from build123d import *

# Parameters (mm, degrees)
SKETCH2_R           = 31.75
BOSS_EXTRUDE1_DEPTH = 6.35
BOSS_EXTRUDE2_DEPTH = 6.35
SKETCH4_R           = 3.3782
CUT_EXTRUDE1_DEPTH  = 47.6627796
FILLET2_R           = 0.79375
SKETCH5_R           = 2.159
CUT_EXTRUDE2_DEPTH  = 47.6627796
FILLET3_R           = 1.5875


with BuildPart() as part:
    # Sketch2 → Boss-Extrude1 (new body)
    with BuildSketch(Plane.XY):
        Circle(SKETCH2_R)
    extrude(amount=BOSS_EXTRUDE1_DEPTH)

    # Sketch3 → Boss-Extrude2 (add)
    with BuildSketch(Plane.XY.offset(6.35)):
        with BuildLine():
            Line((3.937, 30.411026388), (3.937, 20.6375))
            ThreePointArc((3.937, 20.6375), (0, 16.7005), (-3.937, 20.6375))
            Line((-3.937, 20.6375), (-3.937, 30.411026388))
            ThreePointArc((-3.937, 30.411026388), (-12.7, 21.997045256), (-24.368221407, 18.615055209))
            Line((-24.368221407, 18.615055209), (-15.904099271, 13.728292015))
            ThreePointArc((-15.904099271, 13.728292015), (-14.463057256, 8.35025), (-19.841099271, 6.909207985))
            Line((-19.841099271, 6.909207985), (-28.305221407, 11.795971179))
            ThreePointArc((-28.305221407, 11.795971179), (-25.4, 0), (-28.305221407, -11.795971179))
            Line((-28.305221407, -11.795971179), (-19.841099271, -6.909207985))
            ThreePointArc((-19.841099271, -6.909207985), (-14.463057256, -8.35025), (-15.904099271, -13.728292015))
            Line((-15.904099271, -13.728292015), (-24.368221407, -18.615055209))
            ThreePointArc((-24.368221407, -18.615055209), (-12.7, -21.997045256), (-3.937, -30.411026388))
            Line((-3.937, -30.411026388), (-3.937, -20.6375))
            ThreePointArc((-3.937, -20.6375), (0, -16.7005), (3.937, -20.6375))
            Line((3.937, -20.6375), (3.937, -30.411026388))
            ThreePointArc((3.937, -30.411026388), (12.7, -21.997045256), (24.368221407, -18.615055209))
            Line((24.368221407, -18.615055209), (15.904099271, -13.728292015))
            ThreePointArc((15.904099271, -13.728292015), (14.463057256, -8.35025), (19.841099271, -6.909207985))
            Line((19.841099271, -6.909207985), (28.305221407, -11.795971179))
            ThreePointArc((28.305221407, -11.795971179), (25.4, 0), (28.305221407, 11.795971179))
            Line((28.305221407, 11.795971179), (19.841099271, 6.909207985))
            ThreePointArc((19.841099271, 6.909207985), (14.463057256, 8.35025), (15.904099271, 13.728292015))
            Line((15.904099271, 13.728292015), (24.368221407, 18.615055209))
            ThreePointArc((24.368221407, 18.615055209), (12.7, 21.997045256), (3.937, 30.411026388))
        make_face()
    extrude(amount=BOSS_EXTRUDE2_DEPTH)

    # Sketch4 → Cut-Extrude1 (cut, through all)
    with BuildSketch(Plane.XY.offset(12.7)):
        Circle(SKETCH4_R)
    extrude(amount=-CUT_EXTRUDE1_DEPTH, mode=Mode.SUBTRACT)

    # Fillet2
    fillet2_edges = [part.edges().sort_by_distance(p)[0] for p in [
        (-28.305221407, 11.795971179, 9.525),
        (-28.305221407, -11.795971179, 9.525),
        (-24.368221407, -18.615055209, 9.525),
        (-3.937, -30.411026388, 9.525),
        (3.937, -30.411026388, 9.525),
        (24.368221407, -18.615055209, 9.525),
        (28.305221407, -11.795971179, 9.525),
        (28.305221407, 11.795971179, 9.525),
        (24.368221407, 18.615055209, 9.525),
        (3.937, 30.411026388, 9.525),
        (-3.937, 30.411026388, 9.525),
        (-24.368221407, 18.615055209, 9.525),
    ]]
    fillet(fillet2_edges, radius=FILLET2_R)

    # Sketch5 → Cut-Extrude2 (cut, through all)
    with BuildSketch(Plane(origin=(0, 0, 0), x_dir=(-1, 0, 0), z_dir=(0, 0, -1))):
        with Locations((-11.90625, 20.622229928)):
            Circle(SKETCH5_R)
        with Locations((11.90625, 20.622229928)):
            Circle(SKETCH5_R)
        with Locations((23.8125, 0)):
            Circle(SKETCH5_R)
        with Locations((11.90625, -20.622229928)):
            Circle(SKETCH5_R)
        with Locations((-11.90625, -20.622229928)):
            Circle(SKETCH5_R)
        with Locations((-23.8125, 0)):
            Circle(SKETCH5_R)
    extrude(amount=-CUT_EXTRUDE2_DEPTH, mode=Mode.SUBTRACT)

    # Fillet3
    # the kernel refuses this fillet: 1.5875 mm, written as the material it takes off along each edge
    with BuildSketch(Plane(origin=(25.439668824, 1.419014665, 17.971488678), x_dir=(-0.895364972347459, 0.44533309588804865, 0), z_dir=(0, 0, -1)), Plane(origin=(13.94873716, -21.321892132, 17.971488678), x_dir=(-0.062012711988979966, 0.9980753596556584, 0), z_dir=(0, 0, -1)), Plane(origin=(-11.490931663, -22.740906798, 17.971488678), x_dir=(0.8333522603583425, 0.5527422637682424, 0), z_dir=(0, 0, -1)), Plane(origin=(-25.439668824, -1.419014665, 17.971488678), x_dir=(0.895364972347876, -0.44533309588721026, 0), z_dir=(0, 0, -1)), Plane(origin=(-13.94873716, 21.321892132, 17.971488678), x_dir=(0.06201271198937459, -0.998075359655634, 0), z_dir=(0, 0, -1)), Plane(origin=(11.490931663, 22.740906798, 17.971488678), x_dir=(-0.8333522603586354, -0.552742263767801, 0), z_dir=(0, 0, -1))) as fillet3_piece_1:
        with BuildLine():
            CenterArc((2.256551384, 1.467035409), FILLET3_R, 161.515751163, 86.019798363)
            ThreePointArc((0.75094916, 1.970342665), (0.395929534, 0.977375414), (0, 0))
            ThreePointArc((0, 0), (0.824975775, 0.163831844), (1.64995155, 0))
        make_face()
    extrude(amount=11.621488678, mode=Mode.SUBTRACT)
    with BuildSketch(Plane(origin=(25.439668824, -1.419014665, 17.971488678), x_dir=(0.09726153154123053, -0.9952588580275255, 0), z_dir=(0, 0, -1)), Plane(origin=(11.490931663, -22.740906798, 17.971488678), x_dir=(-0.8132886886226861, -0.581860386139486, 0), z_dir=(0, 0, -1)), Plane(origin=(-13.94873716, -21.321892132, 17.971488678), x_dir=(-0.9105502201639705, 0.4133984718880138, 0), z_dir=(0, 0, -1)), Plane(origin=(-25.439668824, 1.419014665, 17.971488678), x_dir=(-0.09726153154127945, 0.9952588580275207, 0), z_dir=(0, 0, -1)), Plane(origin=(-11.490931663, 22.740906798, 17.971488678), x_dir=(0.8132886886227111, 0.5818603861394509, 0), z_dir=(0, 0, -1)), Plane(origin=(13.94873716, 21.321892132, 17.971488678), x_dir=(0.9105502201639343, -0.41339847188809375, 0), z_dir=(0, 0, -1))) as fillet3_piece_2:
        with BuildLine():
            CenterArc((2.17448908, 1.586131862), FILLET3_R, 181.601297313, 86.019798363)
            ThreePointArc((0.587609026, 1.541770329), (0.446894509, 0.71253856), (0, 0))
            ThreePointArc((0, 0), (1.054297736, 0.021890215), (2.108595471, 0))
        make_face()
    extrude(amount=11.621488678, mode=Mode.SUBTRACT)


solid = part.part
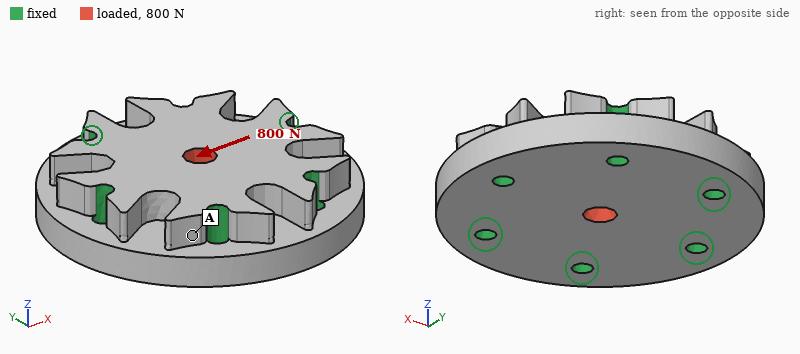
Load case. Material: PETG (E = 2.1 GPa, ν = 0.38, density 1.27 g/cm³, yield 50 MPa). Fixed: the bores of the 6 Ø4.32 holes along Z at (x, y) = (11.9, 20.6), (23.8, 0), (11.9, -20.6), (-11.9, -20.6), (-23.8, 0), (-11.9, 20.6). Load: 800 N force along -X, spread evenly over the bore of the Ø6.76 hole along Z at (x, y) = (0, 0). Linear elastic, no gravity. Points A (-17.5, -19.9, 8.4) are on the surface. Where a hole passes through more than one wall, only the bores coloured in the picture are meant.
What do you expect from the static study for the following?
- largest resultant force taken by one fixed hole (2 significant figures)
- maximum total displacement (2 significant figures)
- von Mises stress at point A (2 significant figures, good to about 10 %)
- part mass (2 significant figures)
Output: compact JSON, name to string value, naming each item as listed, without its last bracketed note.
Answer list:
{"largest resultant force taken by one fixed hole": "220 N", "maximum total displacement": "19 µm", "von Mises stress at point A": "0.63 MPa", "part mass": "38 g"}
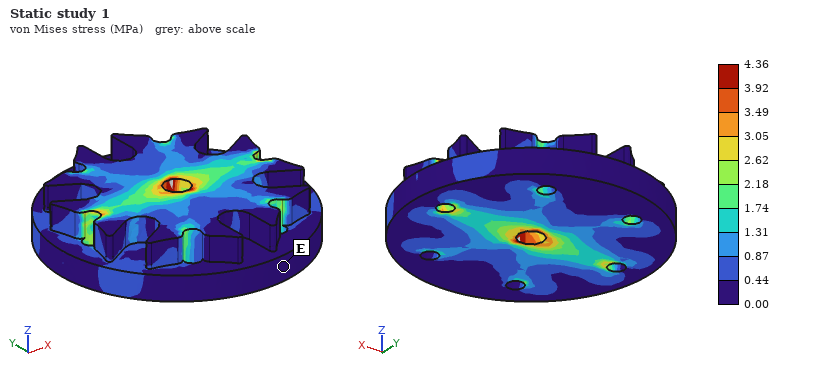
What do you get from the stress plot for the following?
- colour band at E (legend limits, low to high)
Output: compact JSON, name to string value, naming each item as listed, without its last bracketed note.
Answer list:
{"colour band at E": "0.00 to 0.44 MPa"}
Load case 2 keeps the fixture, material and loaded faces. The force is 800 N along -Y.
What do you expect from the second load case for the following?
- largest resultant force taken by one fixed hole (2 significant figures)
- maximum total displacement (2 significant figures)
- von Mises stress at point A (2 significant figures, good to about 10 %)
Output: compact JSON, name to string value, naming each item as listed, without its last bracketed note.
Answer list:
{"largest resultant force taken by one fixed hole": "200 N", "maximum total displacement": "19 µm", "von Mises stress at point A": "0.51 MPa"}
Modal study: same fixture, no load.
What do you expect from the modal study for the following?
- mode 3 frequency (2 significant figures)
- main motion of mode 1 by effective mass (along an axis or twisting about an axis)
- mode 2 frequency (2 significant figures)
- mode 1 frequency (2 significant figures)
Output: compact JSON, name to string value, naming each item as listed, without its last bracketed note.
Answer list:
{"mode 3 frequency": "11 kHz", "main motion of mode 1 by effective mass": "along Z", "mode 2 frequency": "11 kHz", "mode 1 frequency": "7700 Hz"}
